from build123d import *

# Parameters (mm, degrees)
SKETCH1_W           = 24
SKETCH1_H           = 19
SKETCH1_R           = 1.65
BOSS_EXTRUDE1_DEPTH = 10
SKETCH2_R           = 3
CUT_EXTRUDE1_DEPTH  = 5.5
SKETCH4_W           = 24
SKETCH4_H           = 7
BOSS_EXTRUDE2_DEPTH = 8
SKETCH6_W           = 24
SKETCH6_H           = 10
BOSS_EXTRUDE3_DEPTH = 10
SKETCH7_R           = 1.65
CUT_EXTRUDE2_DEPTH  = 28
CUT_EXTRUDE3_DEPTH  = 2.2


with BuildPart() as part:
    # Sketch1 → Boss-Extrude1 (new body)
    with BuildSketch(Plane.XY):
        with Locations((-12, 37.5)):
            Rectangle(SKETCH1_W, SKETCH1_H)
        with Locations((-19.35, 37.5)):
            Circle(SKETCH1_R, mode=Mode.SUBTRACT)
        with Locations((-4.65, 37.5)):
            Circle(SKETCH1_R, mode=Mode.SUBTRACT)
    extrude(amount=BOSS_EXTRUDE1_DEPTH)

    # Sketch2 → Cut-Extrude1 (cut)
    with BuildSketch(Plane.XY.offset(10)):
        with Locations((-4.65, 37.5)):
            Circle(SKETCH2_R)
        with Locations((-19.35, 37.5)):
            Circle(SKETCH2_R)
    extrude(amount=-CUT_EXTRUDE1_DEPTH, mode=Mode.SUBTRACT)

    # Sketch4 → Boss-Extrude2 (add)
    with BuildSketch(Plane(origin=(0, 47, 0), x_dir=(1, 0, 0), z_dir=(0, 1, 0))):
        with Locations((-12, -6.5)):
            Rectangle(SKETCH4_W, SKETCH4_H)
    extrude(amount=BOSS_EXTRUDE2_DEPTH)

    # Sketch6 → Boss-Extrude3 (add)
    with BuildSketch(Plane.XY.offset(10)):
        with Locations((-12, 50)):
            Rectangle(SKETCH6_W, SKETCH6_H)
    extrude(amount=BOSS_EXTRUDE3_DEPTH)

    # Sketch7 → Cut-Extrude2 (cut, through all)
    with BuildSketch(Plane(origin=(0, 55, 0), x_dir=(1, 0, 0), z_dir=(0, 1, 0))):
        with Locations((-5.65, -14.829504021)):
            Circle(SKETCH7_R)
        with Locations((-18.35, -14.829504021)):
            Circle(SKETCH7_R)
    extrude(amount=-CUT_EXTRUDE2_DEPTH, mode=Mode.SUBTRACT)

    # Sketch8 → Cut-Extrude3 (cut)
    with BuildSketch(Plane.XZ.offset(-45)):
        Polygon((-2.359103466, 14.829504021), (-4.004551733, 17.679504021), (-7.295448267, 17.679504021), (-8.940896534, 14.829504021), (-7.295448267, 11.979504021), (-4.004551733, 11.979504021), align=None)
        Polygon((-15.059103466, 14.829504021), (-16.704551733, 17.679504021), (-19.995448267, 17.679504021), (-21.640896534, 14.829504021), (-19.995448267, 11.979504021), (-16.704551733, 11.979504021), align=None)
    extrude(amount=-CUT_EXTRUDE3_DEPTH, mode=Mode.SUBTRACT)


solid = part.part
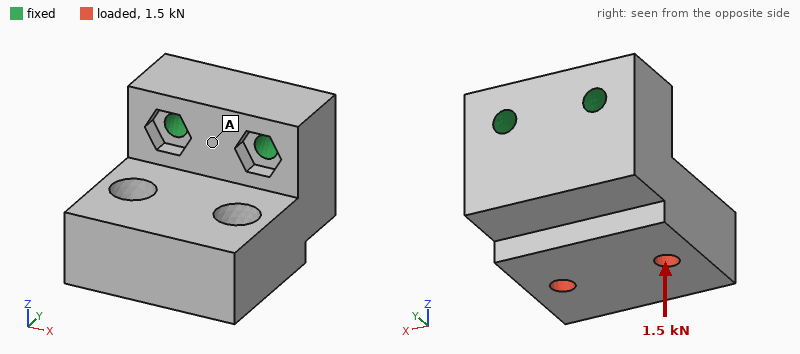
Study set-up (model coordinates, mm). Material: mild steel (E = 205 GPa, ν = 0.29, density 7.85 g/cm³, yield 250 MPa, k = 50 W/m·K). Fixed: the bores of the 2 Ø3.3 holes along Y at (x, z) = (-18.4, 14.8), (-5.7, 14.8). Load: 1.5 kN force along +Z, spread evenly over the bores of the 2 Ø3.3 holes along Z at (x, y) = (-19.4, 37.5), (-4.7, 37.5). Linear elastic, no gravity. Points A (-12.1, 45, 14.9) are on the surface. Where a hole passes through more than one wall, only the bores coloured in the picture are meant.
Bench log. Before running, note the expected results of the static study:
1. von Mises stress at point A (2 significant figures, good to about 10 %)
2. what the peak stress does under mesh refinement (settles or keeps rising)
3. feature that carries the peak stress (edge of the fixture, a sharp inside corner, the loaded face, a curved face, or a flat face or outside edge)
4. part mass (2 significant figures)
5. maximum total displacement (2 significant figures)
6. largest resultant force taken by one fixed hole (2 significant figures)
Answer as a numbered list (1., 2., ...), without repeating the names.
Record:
1. 22 MPa
2. keeps rising
3. edge of the fixture
4. 60 g
5. 22 µm
6. 760 N
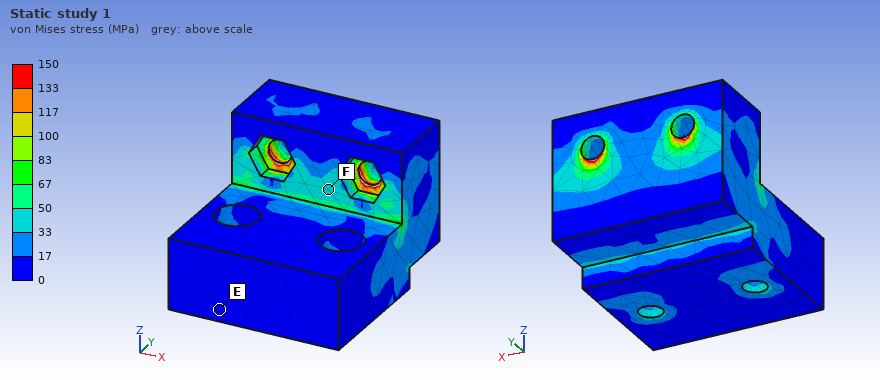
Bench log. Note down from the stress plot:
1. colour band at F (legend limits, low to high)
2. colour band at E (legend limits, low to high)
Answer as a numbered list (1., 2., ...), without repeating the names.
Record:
1. 33 to 50 MPa
2. 0 to 17 MPa
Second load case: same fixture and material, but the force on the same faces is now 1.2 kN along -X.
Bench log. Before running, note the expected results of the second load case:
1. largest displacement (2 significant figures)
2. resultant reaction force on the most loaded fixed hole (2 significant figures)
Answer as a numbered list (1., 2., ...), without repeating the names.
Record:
1. 6.4 µm
2. 1.5 kN
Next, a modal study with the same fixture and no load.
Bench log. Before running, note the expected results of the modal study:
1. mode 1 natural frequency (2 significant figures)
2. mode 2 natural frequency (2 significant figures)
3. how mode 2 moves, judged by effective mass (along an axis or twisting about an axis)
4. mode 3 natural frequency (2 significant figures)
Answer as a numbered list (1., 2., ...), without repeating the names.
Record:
1. 8200 Hz
2. 13 kHz
3. along X
4. 22 kHz
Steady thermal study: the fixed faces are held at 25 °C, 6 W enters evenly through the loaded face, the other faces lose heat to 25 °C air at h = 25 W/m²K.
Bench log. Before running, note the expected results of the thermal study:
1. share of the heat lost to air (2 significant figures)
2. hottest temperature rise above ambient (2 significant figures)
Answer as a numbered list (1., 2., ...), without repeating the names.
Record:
1. 7.6 %
2. 13 K
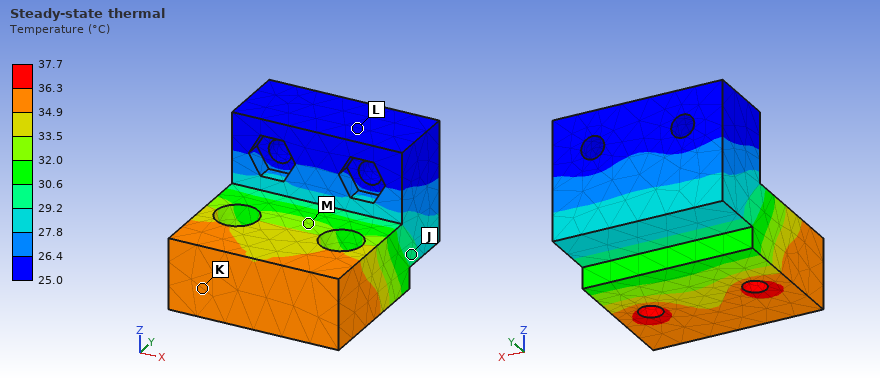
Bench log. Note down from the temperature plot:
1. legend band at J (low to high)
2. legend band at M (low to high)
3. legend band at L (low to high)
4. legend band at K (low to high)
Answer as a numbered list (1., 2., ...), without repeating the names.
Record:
1. 29.2 to 30.6 °C
2. 32.0 to 33.5 °C
3. 25.0 to 26.4 °C
4. 34.9 to 36.3 °C
